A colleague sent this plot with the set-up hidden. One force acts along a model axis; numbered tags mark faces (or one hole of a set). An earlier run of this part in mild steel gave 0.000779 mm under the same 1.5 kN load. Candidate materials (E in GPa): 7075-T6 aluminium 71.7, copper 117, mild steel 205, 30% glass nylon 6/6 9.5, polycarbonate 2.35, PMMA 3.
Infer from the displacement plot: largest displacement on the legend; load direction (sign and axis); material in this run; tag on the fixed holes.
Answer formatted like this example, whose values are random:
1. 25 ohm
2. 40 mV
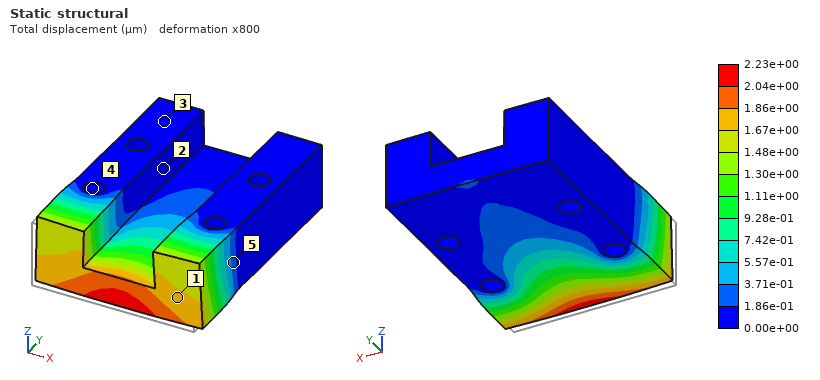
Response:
1. 2.23e+00 µm
2. +Y
3. 7075-T6 aluminium
4. 4
